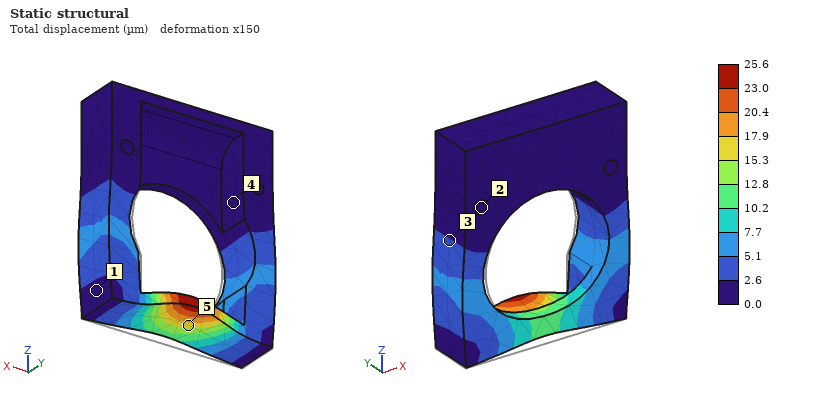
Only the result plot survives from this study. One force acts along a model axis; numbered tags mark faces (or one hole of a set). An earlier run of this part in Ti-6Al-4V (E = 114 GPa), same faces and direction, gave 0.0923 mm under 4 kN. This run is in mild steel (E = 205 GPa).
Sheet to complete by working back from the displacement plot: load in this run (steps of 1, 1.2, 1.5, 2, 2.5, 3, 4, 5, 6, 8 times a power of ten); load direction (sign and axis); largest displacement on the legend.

2 kN
+Z
25.6 µm
